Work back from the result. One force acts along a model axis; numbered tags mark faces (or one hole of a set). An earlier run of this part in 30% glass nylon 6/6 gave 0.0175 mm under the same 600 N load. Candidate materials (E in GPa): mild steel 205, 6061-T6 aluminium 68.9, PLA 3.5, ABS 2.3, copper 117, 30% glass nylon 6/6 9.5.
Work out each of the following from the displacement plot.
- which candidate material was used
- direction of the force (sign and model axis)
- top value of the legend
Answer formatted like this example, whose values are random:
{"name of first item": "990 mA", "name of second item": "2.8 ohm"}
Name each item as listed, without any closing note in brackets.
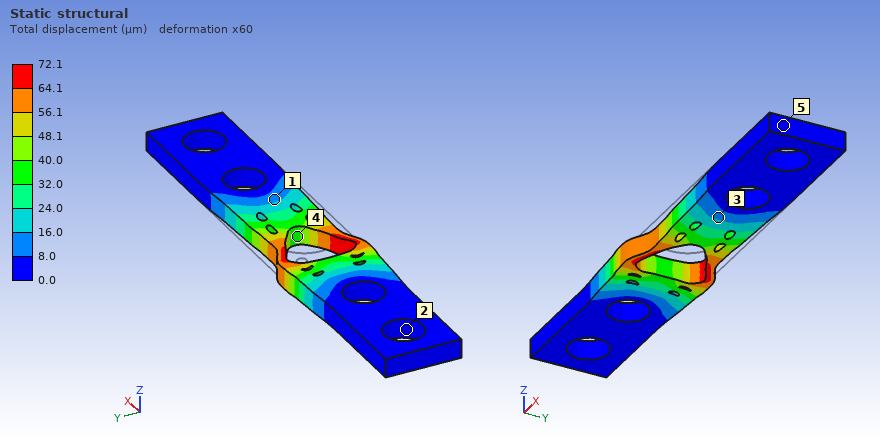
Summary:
{"which candidate material was used": "ABS", "direction of the force": "-X", "top value of the legend": "72.1 µm"}
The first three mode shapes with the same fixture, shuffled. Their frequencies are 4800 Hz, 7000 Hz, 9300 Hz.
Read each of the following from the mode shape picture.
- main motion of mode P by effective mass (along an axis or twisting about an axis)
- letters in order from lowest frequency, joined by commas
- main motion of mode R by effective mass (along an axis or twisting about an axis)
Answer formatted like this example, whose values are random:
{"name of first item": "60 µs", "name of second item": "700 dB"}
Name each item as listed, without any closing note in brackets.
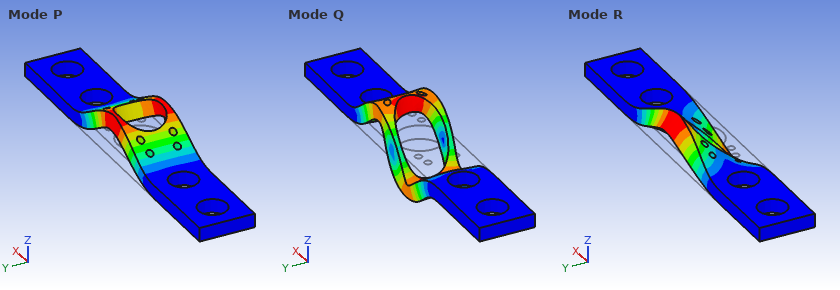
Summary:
{"main motion of mode P by effective mass": "along Z", "letters in order from lowest frequency, joined by commas": "P, R, Q", "main motion of mode R by effective mass": "twisting about X"}
